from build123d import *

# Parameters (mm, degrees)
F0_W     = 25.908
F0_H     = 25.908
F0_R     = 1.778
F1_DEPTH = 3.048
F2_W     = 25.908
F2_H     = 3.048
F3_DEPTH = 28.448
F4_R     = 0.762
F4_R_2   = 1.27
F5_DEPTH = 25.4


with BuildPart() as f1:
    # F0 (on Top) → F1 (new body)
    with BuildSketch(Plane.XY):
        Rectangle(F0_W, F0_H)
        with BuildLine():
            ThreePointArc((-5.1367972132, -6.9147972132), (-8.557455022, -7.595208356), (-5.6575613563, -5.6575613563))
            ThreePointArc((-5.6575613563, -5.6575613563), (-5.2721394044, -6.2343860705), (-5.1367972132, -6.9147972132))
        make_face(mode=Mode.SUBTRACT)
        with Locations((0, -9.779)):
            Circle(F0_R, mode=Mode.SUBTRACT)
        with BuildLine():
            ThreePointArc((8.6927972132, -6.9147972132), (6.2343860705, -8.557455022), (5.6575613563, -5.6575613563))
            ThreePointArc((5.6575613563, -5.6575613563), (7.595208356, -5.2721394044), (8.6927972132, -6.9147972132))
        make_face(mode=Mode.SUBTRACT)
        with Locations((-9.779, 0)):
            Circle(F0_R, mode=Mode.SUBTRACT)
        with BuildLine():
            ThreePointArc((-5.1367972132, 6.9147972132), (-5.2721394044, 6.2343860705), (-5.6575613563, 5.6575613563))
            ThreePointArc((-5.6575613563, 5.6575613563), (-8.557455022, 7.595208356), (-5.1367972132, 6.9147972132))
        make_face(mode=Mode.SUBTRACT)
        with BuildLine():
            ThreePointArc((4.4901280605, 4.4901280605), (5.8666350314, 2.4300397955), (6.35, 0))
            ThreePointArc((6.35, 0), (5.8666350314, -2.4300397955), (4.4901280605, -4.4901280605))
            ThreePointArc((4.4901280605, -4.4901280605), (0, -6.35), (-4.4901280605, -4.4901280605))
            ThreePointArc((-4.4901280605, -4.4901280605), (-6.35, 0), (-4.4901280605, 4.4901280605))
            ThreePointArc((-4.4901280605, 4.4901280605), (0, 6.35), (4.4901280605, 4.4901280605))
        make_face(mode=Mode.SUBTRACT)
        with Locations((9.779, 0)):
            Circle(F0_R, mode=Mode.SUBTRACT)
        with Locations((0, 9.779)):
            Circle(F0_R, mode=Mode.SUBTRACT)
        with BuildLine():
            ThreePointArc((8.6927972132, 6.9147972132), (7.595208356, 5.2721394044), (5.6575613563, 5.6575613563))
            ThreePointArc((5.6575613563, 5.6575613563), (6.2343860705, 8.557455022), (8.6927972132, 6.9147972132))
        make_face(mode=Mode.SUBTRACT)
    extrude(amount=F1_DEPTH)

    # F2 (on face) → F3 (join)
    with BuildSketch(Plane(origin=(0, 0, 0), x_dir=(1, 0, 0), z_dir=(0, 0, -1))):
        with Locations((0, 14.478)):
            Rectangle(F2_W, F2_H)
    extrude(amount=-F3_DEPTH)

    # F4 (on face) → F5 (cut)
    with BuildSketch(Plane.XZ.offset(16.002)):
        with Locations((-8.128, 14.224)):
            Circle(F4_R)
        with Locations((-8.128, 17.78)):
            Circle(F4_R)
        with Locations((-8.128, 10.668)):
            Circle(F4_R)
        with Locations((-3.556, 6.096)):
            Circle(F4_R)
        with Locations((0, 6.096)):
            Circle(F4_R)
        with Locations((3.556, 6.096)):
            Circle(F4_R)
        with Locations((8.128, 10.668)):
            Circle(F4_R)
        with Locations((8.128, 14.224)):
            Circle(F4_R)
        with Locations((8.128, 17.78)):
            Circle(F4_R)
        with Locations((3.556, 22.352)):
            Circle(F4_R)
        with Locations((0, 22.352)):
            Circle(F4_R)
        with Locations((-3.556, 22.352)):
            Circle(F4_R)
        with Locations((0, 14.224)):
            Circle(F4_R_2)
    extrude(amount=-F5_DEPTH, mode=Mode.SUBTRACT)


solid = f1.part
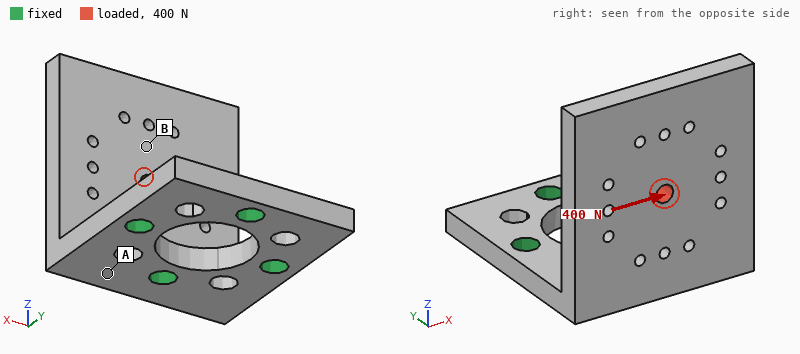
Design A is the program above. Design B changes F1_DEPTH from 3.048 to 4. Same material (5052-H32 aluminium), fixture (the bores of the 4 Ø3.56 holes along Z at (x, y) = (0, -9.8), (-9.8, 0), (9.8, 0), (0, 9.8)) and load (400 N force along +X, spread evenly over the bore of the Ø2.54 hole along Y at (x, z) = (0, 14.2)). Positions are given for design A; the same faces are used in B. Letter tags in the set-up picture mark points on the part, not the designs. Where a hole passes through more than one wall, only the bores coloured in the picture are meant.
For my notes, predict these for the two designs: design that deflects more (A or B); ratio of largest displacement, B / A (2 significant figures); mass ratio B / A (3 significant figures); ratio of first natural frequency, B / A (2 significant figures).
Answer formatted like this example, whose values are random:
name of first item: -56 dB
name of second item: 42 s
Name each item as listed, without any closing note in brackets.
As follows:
design that deflects more: A
ratio of largest displacement, B / A: 0.56
mass ratio B / A: 1.12
ratio of first natural frequency, B / A: 1.2
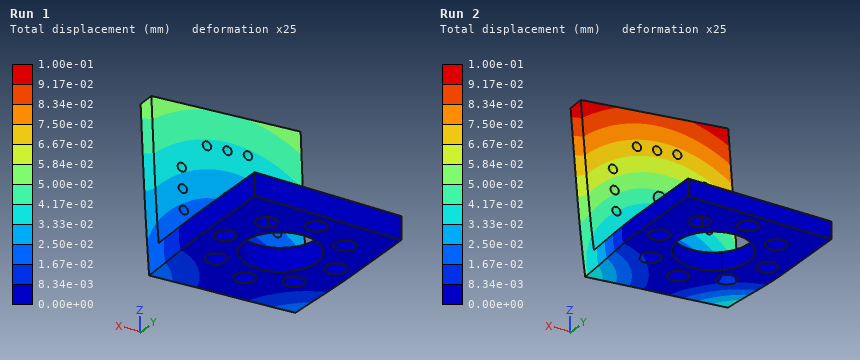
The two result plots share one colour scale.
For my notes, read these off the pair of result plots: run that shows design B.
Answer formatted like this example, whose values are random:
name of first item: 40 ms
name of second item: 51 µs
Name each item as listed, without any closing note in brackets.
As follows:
run that shows design B: Run 1
